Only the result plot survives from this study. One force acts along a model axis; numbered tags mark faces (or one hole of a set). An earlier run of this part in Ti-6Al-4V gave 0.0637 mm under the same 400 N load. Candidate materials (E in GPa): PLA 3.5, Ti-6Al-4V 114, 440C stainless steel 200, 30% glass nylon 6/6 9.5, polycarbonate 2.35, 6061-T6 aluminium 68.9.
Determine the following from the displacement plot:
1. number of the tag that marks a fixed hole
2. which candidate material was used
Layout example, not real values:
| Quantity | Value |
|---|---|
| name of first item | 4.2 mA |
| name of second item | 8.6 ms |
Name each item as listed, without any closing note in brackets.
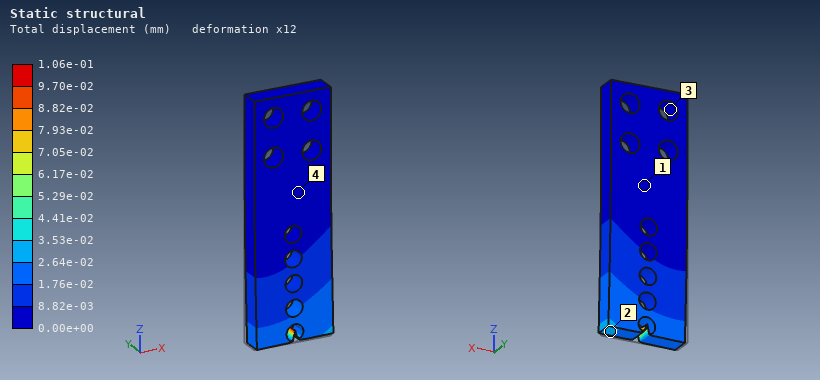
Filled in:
| Quantity | Value |
|---|---|
| number of the tag that marks a fixed hole | 3 |
| which candidate material was used | 6061-T6 aluminium |
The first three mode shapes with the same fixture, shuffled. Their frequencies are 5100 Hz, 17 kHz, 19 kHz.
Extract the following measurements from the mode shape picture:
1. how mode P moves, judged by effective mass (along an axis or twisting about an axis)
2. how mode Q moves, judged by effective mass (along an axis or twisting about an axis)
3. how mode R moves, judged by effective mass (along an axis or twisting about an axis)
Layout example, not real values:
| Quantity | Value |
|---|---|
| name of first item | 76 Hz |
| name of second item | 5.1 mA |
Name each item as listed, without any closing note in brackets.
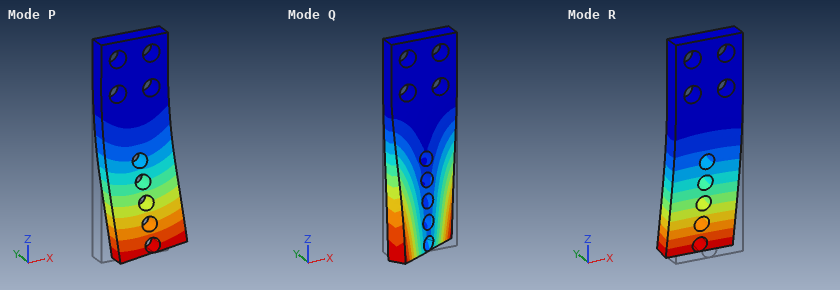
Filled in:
| Quantity | Value |
|---|---|
| how mode P moves, judged by effective mass | along X |
| how mode Q moves, judged by effective mass | twisting about Z |
| how mode R moves, judged by effective mass | along Y |
